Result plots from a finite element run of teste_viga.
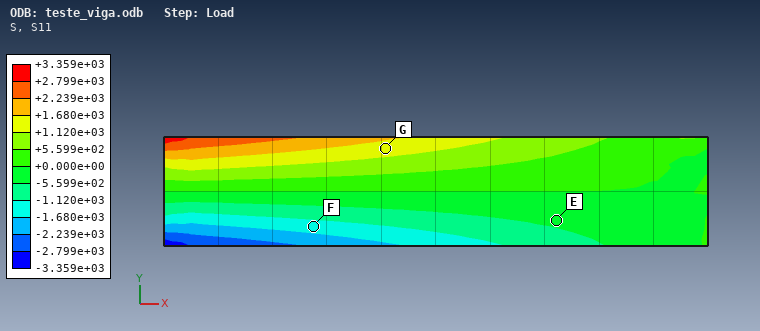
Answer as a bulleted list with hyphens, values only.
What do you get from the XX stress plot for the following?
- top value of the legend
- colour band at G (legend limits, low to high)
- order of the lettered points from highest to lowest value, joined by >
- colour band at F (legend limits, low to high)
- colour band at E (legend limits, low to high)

- +3.359e+03
- +1.120e+03 to +1.680e+03
- G > E > F
- -1.680e+03 to -1.120e+03
- -5.599e+02 to +0.000e+00
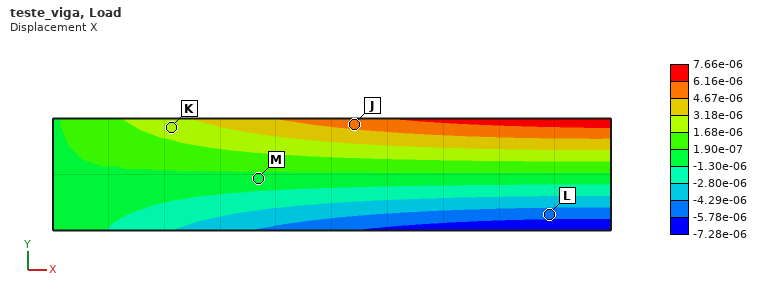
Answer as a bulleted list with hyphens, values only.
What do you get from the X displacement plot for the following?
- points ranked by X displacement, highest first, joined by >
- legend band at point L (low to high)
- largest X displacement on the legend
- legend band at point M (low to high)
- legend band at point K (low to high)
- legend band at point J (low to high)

- J > K > M > L
- -5.78e-06 to -4.29e-06
- 7.66e-06
- -1.30e-06 to 1.90e-07
- 1.68e-06 to 3.18e-06
- 4.67e-06 to 6.16e-06
